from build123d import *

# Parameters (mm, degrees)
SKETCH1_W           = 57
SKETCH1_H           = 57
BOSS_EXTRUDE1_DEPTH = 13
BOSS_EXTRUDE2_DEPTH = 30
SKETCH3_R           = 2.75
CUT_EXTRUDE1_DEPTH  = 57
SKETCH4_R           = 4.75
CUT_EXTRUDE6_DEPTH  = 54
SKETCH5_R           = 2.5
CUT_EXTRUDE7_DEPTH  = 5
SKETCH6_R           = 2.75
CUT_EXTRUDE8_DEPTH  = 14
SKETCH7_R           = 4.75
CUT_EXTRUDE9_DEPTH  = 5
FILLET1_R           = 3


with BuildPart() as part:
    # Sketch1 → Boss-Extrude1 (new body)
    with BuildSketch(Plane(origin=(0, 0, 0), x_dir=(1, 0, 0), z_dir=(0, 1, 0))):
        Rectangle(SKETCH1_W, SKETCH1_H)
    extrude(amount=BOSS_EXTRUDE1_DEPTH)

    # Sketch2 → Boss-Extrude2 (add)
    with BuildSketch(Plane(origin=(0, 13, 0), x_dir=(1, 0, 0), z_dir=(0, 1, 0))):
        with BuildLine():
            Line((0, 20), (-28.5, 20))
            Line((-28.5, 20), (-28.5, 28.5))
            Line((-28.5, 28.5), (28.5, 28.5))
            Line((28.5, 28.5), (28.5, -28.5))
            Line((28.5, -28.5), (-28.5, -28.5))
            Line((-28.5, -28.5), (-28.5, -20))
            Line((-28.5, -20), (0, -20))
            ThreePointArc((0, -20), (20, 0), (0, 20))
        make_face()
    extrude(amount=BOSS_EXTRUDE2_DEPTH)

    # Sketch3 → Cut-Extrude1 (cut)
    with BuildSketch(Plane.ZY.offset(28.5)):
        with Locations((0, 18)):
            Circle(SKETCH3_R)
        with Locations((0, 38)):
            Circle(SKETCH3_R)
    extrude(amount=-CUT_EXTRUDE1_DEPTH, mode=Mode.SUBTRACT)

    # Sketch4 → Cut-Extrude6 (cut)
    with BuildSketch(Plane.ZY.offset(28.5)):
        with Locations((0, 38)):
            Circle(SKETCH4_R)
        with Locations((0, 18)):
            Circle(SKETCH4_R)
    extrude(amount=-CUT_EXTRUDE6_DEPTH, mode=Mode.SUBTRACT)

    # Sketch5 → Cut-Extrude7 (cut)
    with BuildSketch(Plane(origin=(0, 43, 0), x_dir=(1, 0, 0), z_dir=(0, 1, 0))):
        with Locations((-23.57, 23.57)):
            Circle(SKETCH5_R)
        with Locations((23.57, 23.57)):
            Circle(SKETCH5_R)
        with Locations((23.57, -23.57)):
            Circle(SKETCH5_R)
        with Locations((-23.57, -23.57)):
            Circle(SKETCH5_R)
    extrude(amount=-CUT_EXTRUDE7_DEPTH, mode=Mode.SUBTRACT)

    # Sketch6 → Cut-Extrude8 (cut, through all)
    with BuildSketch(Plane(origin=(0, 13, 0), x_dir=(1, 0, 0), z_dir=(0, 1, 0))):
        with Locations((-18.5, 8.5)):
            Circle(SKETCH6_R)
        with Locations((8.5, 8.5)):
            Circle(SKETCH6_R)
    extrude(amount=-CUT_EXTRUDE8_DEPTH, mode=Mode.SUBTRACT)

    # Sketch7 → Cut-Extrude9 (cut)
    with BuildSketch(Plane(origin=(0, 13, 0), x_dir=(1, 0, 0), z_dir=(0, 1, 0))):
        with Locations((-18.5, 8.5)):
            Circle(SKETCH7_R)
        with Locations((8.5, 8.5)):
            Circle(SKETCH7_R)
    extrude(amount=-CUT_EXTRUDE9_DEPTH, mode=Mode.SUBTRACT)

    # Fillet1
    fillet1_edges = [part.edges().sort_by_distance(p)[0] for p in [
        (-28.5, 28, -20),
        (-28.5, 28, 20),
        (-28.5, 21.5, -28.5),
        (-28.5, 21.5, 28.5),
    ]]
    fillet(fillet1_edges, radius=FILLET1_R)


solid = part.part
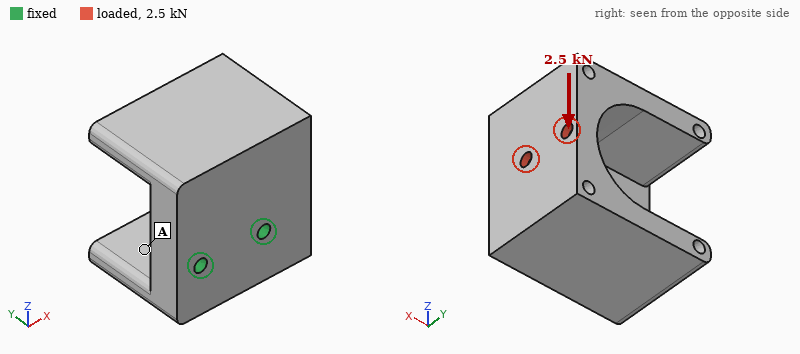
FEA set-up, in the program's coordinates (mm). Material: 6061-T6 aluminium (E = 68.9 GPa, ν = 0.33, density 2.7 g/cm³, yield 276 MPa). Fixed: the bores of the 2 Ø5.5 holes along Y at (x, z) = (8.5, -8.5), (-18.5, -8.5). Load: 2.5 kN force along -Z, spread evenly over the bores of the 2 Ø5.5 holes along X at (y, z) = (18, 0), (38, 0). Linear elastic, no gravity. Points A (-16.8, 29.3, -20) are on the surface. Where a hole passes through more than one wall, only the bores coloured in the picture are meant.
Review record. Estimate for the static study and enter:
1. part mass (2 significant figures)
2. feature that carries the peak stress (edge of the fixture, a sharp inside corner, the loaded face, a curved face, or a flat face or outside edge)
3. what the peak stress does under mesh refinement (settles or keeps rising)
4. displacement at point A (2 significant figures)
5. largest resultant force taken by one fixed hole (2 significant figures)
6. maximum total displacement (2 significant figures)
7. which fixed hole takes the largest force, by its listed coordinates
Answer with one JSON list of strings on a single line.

["230 g", "edge of the fixture", "keeps rising", "0.041 mm", "3.9 kN", "0.11 mm", "(8.5, -8.5)"]
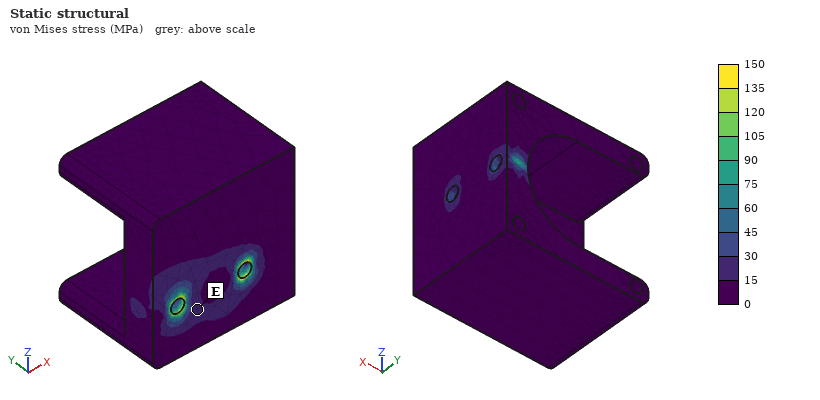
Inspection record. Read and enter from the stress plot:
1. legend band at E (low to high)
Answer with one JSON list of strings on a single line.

["15 to 30 MPa"]
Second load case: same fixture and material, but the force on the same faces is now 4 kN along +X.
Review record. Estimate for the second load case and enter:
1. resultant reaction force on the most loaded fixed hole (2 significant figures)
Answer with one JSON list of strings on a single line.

["3.8 kN"]
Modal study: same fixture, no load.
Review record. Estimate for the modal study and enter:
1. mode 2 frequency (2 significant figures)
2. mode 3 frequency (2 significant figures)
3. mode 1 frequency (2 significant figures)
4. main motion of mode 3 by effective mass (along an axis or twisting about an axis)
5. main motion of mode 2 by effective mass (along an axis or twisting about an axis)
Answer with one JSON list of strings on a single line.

["4500 Hz", "6600 Hz", "2200 Hz", "along Y", "along X"]
